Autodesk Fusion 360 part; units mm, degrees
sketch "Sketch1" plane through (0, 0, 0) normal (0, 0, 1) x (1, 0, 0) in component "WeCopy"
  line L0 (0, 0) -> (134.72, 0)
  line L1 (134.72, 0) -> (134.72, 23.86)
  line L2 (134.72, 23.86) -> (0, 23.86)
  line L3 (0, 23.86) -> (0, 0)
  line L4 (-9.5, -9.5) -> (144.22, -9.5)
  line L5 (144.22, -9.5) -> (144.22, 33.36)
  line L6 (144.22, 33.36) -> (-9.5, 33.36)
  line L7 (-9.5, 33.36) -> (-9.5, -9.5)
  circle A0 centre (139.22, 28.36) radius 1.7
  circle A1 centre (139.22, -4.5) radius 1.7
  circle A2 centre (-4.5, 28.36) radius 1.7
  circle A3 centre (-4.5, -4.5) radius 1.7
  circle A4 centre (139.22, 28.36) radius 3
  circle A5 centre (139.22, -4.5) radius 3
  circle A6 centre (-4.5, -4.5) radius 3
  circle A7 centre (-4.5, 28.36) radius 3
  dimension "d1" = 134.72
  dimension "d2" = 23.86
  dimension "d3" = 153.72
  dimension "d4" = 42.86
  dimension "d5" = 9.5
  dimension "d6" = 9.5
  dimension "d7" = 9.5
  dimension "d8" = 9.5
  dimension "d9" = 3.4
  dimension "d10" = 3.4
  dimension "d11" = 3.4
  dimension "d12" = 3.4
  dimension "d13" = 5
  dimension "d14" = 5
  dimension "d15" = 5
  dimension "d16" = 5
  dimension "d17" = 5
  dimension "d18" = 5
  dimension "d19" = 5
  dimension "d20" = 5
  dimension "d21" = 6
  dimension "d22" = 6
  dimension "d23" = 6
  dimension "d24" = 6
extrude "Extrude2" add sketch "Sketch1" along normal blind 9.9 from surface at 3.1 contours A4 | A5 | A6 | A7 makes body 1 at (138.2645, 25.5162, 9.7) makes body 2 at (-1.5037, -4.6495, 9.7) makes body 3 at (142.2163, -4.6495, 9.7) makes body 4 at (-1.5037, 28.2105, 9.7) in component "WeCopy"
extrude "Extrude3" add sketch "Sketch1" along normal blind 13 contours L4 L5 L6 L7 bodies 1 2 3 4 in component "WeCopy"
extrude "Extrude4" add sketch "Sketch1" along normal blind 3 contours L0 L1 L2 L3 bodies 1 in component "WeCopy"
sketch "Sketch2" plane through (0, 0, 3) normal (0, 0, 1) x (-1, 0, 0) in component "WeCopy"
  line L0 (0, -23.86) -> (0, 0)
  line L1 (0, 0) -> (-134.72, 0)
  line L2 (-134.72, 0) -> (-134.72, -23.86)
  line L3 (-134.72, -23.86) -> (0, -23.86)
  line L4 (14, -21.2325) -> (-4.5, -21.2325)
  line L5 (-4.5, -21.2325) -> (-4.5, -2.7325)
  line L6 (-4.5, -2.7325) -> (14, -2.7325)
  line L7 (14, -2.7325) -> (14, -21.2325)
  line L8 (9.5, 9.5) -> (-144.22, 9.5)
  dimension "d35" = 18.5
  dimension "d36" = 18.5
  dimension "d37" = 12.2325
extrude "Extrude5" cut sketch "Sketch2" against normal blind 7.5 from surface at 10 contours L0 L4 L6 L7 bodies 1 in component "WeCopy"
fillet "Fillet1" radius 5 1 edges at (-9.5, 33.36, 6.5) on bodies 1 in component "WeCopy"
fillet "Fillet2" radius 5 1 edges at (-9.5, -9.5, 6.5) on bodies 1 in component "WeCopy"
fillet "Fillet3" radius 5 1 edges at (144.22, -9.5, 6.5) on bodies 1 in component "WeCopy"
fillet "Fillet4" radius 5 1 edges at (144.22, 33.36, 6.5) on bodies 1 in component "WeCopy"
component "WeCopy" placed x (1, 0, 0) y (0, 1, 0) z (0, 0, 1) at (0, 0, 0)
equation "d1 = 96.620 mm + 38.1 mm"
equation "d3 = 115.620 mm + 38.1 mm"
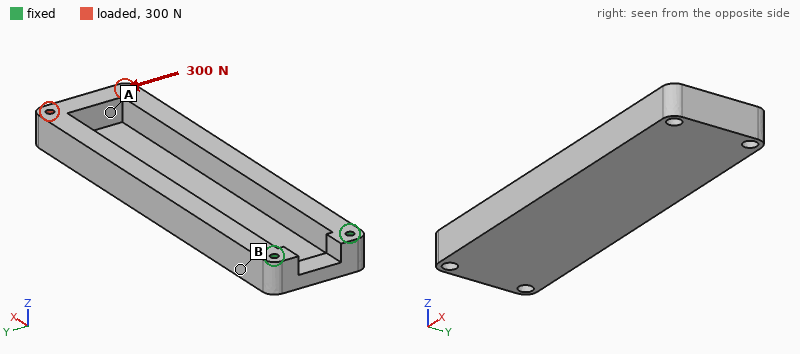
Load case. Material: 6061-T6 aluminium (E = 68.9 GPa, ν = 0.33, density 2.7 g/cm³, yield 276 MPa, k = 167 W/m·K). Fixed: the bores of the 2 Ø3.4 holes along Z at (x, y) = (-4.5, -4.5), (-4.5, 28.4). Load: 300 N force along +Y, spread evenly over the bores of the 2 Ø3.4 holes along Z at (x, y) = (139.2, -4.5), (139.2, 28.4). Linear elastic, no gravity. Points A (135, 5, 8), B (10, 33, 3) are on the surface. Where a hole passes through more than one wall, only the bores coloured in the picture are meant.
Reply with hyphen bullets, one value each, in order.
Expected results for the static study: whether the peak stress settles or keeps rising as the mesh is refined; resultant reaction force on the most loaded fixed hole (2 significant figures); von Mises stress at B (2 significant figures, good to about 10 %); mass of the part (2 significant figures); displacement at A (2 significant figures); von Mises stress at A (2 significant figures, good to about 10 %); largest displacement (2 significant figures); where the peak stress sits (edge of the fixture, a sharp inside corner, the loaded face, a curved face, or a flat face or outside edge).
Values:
- keeps rising
- 1.2 kN
- 14 MPa
- 140 g
- 0.10 mm
- 4.5 MPa
- 0.14 mm
- edge of the fixture
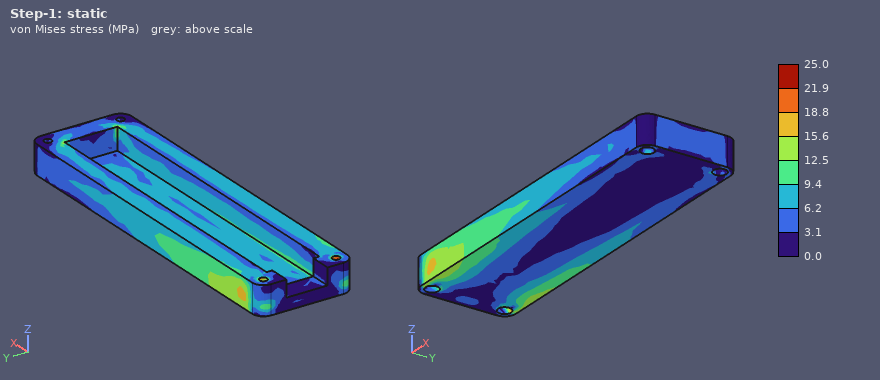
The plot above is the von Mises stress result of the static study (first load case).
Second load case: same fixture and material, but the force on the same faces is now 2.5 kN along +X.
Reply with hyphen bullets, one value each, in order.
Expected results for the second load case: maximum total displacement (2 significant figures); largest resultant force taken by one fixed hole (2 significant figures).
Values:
- 0.21 mm
- 1.3 kN
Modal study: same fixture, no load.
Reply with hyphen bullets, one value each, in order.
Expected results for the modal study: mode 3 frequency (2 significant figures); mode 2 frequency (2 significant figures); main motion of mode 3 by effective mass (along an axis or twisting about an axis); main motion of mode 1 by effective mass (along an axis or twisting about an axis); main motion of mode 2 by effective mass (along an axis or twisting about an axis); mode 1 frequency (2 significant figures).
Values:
- 1900 Hz
- 1200 Hz
- along Y
- along Z
- along Y
- 430 Hz
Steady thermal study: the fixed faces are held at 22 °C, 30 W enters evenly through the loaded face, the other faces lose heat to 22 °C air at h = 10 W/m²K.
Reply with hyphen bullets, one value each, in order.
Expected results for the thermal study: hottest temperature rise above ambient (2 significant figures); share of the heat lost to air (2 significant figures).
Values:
- 70 K
- 24 %
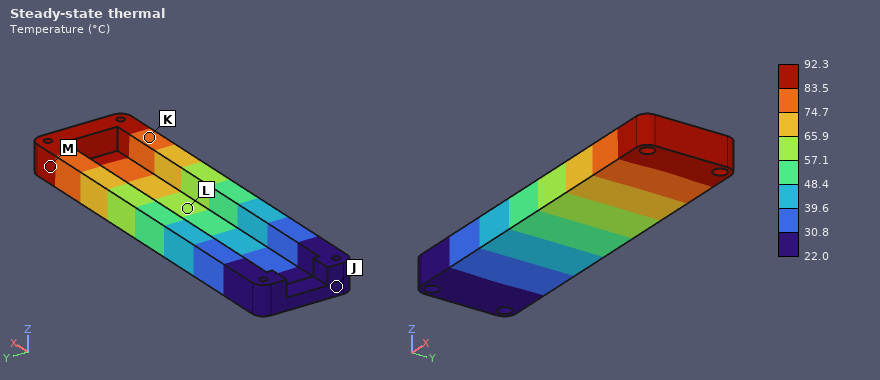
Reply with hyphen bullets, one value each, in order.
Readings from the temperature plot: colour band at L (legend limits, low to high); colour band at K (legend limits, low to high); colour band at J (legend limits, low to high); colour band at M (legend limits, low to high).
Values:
- 57.1 to 65.9 °C
- 74.7 to 83.5 °C
- 22.0 to 30.8 °C
- 83.5 to 92.3 °C
